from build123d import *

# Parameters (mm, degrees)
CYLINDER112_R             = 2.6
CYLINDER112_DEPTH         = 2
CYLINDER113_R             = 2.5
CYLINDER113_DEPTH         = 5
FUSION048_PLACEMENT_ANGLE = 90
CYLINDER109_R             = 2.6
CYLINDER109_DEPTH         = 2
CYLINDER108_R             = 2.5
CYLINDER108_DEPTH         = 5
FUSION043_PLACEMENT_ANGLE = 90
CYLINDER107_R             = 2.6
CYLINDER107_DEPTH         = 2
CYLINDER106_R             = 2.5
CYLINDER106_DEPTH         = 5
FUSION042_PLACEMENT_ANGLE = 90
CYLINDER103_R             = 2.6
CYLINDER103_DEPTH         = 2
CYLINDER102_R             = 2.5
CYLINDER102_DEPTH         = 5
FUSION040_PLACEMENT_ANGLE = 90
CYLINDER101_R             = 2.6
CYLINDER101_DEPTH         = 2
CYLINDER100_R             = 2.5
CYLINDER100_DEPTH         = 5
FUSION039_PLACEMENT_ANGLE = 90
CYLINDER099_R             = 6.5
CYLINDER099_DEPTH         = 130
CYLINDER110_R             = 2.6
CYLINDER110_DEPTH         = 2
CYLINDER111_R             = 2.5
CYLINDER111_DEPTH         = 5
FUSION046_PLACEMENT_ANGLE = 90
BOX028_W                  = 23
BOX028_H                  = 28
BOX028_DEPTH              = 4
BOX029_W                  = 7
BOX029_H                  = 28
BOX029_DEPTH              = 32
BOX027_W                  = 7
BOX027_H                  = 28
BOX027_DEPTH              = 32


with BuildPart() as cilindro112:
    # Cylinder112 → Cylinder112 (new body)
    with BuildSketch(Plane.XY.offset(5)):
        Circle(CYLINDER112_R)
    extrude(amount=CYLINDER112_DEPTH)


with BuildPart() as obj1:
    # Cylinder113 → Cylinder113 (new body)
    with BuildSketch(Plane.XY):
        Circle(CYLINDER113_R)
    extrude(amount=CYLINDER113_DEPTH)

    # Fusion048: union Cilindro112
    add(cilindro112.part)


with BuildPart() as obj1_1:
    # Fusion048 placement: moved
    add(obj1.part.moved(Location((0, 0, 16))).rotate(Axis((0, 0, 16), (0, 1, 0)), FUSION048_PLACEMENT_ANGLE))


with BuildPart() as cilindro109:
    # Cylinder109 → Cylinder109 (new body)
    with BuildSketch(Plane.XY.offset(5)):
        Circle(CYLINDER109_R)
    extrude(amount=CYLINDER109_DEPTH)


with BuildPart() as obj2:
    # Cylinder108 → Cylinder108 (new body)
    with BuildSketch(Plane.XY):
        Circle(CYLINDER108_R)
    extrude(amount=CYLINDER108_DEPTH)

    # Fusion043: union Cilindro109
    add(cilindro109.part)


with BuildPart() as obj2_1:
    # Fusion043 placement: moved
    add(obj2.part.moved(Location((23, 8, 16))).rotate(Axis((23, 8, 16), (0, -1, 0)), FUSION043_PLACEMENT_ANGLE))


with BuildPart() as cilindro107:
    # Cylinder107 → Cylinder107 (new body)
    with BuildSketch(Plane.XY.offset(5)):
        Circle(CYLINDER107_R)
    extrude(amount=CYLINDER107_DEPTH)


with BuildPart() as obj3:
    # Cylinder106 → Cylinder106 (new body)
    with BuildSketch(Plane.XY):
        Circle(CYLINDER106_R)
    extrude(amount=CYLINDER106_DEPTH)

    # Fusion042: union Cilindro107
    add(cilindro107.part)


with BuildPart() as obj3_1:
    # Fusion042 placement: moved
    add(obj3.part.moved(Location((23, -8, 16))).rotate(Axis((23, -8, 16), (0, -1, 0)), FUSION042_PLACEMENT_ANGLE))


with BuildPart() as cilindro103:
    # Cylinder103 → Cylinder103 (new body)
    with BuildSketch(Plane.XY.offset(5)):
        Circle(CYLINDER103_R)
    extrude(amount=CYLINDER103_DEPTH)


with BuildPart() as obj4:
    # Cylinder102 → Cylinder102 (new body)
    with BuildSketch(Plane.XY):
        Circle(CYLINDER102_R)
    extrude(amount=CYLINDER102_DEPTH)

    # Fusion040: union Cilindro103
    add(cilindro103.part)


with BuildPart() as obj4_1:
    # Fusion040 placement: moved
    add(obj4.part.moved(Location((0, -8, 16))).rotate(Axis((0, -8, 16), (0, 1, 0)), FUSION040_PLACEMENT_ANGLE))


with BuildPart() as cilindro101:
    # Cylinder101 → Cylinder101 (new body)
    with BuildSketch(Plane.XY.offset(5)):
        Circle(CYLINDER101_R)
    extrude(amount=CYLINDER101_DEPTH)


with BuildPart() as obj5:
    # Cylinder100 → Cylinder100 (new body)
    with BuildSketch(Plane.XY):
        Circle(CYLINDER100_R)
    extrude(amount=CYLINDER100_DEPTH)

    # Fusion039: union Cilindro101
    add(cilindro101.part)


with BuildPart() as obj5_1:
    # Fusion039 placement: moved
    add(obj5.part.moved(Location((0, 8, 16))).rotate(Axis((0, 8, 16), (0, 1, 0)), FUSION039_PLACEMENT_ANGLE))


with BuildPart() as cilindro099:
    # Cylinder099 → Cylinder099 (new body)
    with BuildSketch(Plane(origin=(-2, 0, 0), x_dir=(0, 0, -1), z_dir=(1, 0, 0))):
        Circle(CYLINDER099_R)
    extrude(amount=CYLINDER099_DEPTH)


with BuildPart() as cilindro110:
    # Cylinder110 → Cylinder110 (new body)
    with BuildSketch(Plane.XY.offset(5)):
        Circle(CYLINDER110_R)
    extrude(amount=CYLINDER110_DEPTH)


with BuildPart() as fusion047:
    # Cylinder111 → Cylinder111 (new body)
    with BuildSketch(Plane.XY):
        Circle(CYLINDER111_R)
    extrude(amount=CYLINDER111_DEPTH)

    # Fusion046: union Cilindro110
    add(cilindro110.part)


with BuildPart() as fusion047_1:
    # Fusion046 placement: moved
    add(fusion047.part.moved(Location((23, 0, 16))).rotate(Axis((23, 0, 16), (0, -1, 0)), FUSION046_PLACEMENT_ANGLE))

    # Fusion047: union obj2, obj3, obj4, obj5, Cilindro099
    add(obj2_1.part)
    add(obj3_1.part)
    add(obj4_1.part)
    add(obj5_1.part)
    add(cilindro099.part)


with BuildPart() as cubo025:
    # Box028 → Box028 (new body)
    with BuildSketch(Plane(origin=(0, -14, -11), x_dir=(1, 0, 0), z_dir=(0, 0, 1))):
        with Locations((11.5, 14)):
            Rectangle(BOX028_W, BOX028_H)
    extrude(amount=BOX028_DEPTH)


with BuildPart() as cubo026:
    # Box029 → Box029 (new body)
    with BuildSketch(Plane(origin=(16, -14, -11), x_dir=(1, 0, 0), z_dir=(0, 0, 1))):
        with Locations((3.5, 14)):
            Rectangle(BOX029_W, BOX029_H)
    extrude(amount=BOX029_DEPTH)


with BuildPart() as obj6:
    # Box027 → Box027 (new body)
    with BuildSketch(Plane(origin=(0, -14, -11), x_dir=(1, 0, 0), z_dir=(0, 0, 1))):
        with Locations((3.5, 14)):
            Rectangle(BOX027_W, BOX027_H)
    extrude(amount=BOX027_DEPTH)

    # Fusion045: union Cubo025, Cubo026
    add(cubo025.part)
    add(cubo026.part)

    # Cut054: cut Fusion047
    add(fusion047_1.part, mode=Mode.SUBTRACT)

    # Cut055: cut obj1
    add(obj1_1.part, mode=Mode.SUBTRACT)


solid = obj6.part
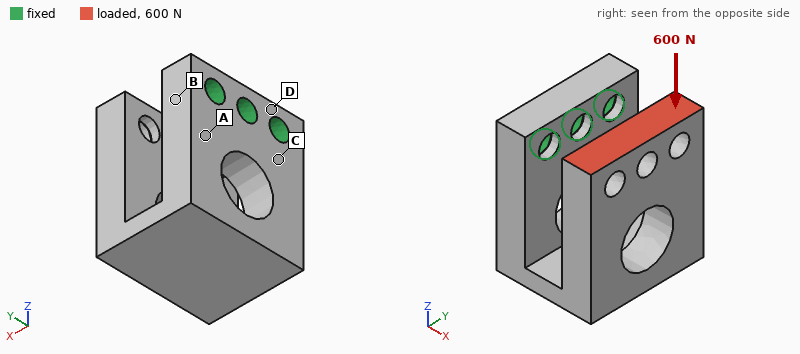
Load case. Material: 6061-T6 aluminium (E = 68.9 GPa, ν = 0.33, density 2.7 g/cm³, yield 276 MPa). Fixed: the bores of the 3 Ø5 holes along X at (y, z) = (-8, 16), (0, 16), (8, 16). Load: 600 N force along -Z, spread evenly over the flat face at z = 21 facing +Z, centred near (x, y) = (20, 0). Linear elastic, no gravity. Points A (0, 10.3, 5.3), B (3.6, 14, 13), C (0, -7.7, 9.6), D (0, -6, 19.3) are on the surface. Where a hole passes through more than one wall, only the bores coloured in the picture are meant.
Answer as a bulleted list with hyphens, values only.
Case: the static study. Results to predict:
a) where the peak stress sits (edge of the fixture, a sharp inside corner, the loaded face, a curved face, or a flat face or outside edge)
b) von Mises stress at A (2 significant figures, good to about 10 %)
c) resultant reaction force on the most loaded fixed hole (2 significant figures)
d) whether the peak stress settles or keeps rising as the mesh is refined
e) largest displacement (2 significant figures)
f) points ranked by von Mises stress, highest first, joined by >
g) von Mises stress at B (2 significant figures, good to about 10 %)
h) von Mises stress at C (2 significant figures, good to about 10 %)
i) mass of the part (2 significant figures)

- edge of the fixture
- 59 MPa
- 280 N
- keeps rising
- 0.35 mm
- A > C > B > D
- 18 MPa
- 45 MPa
- 29 g
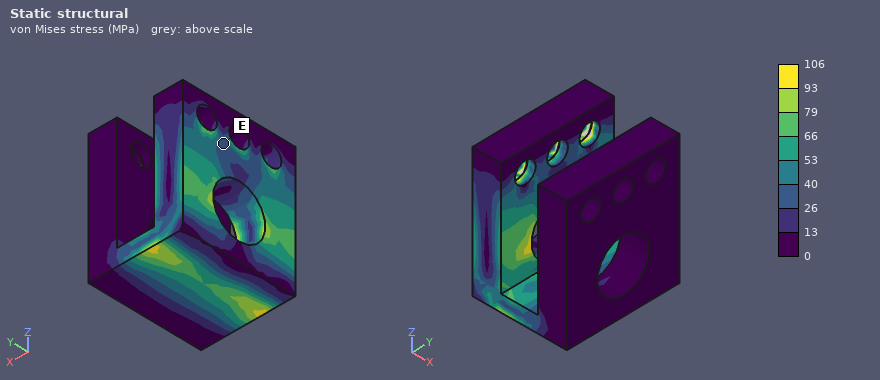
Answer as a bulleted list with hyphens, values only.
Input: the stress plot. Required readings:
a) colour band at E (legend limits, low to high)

- 26 to 40 MPa
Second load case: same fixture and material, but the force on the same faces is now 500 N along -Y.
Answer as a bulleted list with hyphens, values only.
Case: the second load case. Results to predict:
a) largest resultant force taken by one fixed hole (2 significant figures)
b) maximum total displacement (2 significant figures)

- 400 N
- 0.33 mm
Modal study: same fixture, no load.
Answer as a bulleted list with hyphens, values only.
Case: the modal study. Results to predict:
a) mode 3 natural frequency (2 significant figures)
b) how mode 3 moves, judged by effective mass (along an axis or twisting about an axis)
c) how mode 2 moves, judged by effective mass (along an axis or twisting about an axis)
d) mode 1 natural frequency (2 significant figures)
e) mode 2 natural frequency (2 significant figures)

- 3300 Hz
- along X
- along Y
- 1700 Hz
- 2500 Hz
